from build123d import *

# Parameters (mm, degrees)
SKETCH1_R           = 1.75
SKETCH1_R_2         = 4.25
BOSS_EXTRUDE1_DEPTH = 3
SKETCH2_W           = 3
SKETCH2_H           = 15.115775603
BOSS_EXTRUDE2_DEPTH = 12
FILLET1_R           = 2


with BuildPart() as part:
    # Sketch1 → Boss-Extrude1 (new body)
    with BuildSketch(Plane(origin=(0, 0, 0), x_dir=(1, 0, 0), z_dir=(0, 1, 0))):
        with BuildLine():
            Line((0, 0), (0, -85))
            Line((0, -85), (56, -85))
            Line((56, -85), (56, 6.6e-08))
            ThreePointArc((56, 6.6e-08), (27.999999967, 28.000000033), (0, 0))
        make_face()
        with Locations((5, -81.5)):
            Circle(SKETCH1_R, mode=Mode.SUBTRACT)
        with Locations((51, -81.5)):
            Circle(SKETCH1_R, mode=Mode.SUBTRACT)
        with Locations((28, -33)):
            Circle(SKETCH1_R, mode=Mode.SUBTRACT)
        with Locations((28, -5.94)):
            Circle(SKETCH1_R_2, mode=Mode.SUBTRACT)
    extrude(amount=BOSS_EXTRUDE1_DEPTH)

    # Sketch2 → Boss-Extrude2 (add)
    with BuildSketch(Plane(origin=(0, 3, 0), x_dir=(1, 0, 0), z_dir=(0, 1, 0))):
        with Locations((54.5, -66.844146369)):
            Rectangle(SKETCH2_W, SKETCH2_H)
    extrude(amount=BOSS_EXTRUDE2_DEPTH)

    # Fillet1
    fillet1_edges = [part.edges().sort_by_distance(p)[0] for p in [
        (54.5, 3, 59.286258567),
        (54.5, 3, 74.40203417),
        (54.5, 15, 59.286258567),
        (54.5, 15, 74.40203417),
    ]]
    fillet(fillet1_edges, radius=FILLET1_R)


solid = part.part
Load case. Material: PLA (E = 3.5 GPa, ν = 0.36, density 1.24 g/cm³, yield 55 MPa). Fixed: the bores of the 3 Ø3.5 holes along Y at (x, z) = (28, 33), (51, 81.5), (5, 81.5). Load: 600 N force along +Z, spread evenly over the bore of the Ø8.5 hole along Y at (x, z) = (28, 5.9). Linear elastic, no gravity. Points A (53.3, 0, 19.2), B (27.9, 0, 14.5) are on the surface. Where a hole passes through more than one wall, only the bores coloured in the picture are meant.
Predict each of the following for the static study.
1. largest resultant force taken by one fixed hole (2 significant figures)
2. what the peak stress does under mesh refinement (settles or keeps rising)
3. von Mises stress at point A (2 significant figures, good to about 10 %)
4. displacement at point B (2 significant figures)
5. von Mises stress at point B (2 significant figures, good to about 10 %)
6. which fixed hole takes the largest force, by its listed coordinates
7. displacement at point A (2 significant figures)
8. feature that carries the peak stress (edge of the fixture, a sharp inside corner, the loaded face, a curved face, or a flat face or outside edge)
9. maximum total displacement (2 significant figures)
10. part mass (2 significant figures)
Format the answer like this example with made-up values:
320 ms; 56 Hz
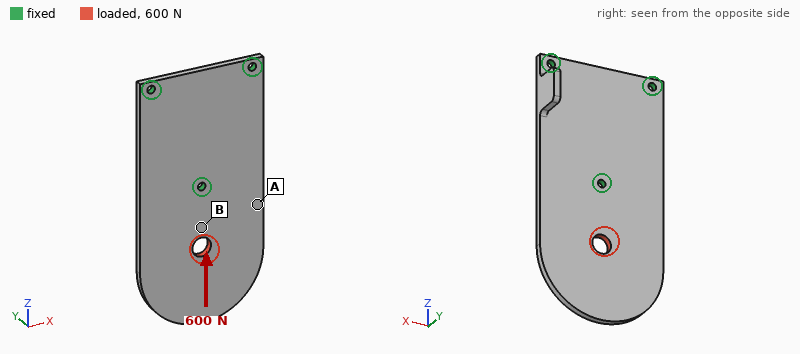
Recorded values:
430 N; keeps rising; 1.1 MPa; 46 µm; 8.1 MPa; (28, 33); 36 µm; edge of the fixture; 75 µm; 23 g
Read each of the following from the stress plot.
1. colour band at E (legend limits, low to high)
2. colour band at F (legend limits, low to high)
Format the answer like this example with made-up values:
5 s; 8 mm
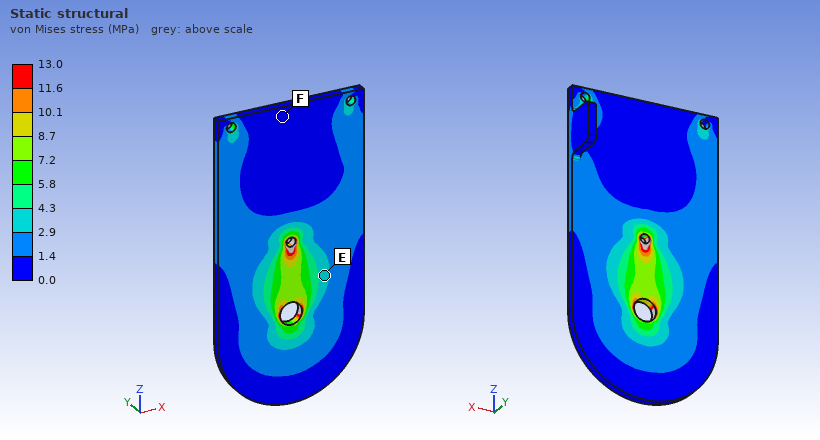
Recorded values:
2.9 to 4.3 MPa; 0.0 to 1.4 MPa
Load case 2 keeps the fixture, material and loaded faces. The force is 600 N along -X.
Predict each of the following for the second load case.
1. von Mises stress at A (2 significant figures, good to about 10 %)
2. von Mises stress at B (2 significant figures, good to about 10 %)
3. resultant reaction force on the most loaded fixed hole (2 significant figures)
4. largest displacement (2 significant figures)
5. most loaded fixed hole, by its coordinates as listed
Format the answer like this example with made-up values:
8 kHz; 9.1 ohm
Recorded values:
5.6 MPa; 10 MPa; 780 N; 0.43 mm; (28, 33)
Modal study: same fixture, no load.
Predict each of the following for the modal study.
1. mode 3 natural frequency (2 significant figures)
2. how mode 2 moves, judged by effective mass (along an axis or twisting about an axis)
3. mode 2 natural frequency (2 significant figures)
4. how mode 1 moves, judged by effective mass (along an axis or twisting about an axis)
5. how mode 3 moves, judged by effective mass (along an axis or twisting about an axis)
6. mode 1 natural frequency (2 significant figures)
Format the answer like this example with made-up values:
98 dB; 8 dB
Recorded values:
1100 Hz; twisting about Z; 490 Hz; along Y; along Y; 240 Hz
